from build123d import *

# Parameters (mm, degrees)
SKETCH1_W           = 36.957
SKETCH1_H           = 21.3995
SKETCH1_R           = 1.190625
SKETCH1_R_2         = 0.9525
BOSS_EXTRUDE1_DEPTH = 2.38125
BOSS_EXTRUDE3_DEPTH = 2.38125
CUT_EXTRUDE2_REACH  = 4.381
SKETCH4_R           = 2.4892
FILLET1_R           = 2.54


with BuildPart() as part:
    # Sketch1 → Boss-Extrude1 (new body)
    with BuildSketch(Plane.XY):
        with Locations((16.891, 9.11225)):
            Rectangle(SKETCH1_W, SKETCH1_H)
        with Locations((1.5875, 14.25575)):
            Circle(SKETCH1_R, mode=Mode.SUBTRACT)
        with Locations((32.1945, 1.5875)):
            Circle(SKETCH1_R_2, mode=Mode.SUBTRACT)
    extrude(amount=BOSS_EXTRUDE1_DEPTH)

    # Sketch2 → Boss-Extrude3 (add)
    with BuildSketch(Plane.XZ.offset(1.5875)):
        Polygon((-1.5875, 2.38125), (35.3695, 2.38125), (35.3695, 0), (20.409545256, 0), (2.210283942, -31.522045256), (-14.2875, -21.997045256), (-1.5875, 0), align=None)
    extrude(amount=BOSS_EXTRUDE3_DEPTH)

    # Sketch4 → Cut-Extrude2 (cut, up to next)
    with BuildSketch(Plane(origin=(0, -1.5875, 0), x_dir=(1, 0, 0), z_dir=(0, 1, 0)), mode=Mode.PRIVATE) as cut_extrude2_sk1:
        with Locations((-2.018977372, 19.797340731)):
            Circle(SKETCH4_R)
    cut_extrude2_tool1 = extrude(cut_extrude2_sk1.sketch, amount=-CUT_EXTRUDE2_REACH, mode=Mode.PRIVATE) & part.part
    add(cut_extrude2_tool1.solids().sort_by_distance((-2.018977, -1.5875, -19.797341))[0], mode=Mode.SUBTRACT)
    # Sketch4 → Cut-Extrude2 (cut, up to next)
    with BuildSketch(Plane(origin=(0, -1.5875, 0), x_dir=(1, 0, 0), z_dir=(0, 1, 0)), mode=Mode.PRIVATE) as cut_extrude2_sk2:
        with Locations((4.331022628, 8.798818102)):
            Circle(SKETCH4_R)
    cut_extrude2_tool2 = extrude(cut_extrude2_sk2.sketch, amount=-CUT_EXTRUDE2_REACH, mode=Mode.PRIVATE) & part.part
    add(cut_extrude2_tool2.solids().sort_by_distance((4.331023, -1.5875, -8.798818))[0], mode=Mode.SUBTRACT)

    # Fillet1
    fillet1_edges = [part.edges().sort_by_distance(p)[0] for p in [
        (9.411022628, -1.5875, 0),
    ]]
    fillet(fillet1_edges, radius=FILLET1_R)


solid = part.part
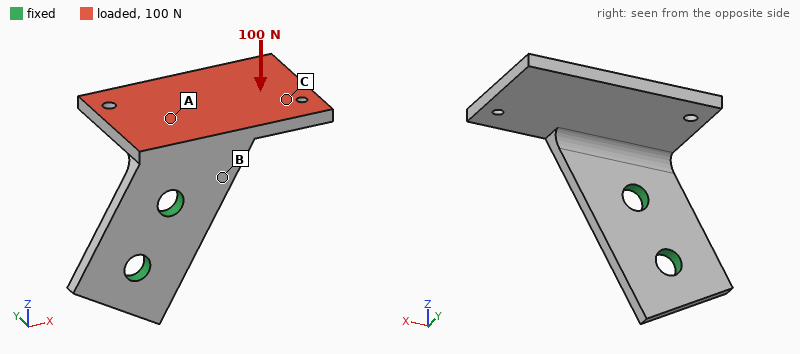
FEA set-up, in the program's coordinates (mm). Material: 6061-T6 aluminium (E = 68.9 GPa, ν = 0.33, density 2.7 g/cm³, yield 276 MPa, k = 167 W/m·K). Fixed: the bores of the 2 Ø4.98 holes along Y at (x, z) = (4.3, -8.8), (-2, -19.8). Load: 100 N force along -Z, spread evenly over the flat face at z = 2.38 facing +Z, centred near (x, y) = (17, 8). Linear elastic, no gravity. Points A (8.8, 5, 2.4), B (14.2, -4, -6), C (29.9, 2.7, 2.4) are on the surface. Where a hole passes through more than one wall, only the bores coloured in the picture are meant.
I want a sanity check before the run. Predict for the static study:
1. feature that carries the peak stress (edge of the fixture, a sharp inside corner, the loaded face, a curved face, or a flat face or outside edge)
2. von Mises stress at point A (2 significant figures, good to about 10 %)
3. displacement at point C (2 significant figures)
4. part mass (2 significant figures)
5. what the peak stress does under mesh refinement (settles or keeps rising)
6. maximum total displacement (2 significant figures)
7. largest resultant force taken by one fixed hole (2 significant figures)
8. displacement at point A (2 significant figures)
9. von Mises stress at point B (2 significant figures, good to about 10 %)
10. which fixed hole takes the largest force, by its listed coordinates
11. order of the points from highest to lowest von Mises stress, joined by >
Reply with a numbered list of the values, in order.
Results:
1. edge of the fixture
2. 22 MPa
3. 0.095 mm
4. 9.2 g
5. keeps rising
6. 0.25 mm
7. 120 N
8. 0.061 mm
9. 41 MPa
10. (4.3, -8.8)
11. B > A > C
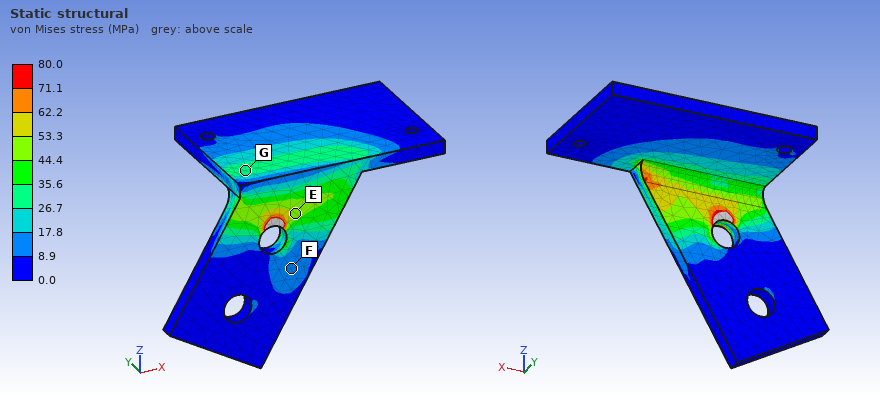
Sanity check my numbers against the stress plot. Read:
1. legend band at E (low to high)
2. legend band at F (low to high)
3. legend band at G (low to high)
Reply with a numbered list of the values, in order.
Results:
1. 44.4 to 53.3 MPa
2. 8.9 to 17.8 MPa
3. 26.7 to 35.6 MPa
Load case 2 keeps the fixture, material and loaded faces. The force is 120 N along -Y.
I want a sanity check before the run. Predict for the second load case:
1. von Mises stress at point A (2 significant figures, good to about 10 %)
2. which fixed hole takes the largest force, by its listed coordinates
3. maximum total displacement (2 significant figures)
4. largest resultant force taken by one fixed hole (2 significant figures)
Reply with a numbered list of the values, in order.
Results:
1. 11 MPa
2. (4.3, -8.8)
3. 0.23 mm
4. 140 N
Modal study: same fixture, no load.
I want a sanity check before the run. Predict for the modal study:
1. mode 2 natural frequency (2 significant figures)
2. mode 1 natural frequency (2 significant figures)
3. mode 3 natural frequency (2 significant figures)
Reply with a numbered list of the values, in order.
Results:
1. 2400 Hz
2. 1600 Hz
3. 4100 Hz
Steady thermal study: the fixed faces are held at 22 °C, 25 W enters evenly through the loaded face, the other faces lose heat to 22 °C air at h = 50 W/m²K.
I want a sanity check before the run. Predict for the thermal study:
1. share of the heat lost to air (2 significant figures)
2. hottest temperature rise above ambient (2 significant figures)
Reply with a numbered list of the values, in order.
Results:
1. 12 %
2. 57 K
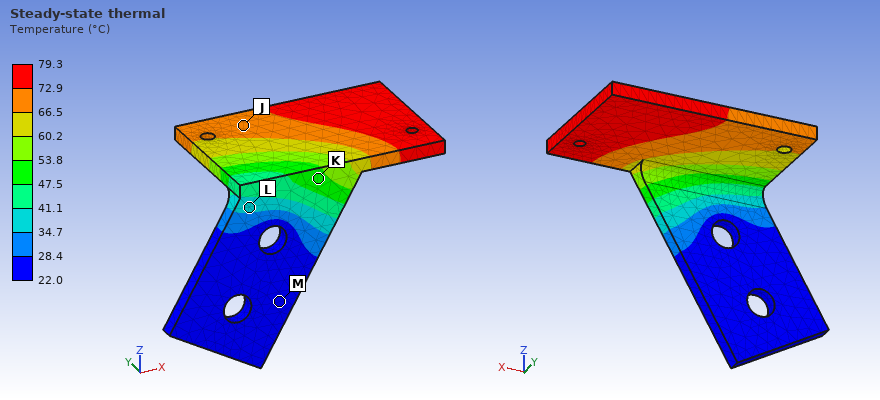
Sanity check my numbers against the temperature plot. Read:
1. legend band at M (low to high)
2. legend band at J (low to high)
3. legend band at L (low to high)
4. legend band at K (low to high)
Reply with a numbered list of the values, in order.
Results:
1. 22.0 to 28.4 °C
2. 66.5 to 72.9 °C
3. 34.7 to 41.1 °C
4. 47.5 to 53.8 °C
